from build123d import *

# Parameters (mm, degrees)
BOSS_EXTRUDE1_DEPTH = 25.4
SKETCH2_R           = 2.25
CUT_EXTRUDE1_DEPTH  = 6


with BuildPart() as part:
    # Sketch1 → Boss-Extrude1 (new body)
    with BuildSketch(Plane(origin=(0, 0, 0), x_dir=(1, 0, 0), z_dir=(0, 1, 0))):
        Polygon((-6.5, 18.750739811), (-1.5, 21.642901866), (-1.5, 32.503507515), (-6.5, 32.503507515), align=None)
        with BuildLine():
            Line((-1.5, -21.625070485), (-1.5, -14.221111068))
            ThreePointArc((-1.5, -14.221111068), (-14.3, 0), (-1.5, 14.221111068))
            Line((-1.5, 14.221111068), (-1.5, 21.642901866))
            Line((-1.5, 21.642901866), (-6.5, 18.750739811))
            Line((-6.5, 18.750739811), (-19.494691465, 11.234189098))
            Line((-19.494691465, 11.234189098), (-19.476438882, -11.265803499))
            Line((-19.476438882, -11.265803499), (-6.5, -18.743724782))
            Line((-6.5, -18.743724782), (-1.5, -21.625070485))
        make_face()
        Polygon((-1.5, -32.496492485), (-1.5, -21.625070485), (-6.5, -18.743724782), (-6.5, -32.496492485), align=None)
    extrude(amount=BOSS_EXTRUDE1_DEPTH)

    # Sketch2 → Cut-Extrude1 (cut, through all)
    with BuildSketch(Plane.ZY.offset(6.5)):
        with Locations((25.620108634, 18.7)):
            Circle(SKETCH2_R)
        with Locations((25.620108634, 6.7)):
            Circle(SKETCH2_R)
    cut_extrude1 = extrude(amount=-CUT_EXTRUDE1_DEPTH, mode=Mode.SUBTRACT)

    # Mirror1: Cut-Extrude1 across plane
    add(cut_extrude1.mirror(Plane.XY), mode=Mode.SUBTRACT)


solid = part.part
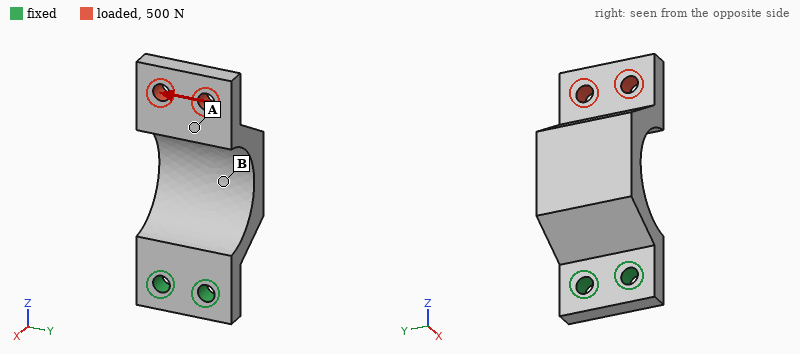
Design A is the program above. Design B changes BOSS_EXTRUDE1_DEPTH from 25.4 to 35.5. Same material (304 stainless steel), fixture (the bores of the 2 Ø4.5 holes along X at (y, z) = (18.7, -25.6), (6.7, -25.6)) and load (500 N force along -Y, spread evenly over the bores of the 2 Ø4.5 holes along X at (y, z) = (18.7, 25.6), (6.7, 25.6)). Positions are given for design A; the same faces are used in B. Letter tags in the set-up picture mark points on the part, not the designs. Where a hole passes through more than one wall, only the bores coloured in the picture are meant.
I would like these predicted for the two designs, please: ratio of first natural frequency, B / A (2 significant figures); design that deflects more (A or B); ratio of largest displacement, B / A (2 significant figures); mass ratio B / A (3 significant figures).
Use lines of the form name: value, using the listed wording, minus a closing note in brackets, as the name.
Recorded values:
ratio of first natural frequency, B / A: 0.95
design that deflects more: A
ratio of largest displacement, B / A: 0.69
mass ratio B / A: 1.41
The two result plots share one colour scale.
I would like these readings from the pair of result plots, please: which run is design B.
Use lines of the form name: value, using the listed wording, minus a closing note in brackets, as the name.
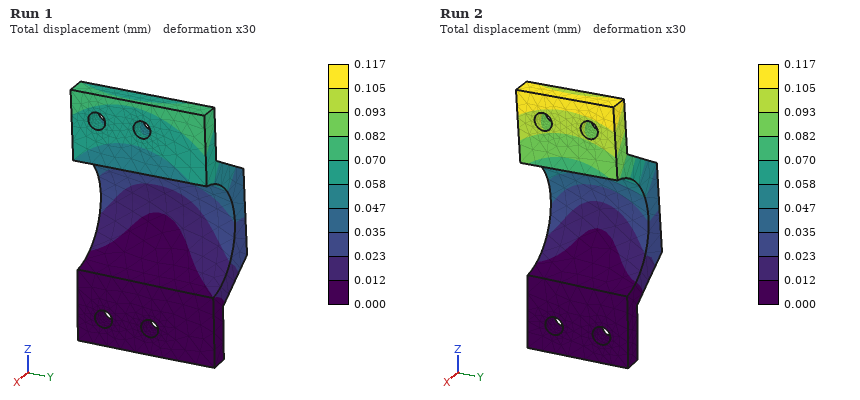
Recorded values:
which run is design B: Run 1
